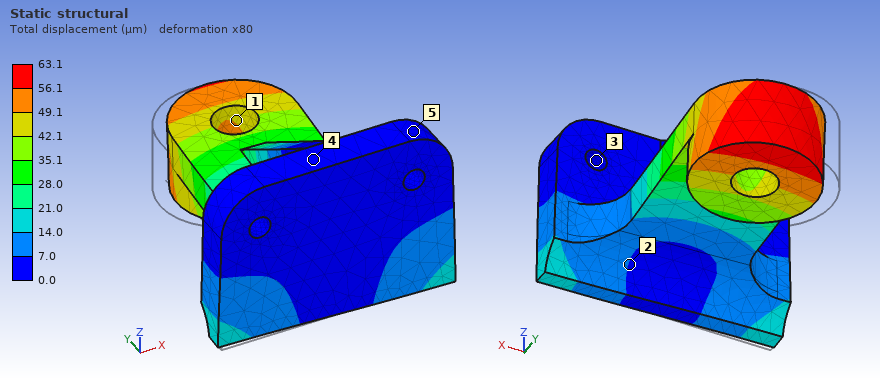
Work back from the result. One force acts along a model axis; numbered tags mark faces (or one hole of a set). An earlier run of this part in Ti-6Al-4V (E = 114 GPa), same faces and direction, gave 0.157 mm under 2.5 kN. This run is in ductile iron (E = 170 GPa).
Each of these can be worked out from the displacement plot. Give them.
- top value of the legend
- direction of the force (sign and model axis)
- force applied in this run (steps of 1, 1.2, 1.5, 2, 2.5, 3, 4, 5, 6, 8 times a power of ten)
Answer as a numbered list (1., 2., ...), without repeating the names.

1. 63.1 µm
2. +X
3. 1.5 kN
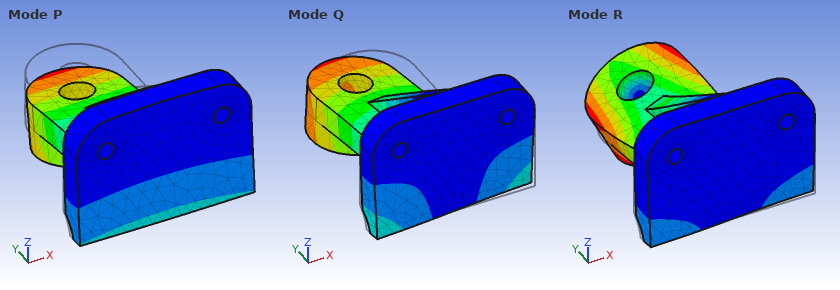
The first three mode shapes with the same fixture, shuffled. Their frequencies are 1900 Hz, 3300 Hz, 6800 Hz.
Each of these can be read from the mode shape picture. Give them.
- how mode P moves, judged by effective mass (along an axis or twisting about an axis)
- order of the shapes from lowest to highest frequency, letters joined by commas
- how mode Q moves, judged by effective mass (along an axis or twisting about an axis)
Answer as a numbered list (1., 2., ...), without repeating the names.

1. along Z
2. P, Q, R
3. along X
